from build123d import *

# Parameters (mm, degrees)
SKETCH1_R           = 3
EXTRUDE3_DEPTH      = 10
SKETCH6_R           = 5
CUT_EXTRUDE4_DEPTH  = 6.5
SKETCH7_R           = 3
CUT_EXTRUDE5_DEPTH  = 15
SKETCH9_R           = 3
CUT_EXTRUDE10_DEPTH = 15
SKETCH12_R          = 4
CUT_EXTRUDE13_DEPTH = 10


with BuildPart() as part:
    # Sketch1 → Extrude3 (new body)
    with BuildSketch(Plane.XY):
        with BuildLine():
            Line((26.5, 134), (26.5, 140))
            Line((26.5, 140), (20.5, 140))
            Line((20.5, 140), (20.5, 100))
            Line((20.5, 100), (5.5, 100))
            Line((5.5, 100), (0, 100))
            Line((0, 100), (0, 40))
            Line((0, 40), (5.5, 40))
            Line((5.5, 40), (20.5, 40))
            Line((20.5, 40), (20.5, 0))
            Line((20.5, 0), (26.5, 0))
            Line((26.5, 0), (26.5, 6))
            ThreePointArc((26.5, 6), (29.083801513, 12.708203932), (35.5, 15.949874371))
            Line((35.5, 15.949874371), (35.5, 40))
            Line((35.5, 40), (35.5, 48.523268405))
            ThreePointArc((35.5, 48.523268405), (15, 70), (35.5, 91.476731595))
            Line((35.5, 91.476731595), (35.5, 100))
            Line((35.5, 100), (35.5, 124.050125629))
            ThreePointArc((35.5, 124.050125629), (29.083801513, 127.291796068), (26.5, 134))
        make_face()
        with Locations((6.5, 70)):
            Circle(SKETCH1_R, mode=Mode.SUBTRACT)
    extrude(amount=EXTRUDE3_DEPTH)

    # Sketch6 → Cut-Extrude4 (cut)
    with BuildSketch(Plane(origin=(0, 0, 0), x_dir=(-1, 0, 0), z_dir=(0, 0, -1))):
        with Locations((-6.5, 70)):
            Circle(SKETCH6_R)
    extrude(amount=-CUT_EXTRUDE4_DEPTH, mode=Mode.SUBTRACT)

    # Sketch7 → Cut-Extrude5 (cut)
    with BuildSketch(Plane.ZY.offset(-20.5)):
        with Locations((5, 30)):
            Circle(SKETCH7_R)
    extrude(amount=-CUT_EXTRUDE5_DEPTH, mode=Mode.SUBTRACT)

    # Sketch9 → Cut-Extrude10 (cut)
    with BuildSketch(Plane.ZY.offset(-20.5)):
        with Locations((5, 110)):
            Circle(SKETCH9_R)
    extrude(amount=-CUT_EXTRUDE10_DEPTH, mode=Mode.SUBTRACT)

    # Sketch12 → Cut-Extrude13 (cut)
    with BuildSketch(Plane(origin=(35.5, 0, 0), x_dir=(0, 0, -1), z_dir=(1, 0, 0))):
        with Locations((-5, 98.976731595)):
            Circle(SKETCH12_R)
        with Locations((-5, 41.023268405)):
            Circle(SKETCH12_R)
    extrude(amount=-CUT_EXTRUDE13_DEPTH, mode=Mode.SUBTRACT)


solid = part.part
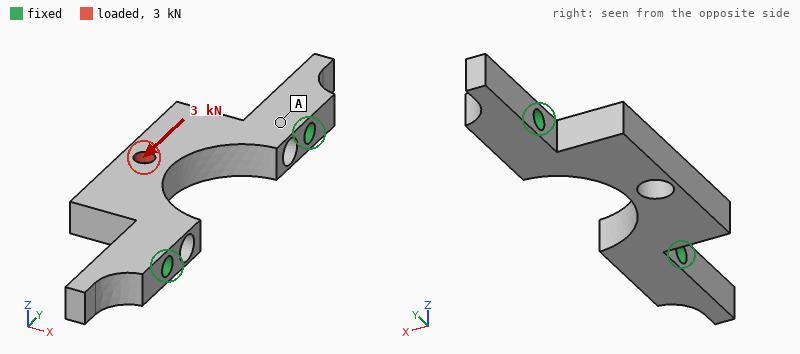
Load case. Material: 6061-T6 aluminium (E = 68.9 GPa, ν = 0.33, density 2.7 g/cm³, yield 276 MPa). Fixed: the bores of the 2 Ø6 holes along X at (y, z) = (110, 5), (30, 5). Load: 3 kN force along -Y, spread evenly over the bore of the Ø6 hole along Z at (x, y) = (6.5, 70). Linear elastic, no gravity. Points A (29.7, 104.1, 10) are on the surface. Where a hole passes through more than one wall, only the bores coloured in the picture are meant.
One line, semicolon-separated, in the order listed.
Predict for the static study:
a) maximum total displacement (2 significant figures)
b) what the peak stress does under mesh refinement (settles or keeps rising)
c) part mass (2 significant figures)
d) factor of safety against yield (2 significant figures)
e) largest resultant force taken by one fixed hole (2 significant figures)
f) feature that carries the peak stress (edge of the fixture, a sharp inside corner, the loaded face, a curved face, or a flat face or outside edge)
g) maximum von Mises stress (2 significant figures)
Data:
21 µm; settles; 58 g; 2.8; 1.7 kN; the loaded face; 100 MPa
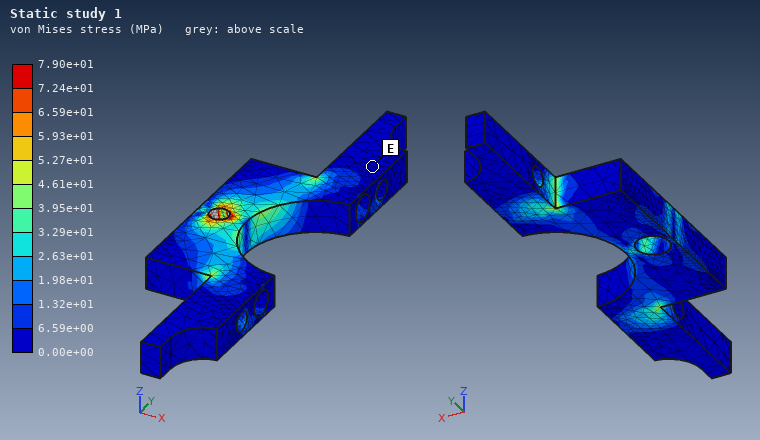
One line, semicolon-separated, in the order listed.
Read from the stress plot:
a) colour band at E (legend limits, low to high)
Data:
0.00e+00 to 6.59e+00 MPa
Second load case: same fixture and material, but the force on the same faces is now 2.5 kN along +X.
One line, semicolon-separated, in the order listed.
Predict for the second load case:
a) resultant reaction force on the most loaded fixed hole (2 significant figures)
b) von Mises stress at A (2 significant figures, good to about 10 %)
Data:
1.9 kN; 37 MPa
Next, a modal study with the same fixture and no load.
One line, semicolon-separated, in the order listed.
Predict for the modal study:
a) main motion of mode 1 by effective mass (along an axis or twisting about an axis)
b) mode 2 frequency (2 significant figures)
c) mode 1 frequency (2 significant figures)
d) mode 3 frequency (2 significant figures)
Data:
along Z; 8600 Hz; 3800 Hz; 11 kHz
